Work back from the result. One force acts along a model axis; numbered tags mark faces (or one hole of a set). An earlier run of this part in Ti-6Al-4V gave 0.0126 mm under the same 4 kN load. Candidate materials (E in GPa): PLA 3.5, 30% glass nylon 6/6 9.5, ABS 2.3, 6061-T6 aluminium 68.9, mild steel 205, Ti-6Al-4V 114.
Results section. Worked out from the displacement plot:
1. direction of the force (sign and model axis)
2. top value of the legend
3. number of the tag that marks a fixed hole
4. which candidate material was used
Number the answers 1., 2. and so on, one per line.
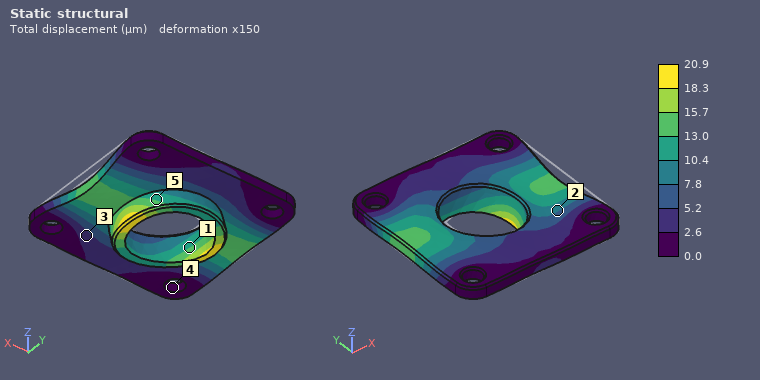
1. -X
2. 20.9 µm
3. 4
4. 6061-T6 aluminium
